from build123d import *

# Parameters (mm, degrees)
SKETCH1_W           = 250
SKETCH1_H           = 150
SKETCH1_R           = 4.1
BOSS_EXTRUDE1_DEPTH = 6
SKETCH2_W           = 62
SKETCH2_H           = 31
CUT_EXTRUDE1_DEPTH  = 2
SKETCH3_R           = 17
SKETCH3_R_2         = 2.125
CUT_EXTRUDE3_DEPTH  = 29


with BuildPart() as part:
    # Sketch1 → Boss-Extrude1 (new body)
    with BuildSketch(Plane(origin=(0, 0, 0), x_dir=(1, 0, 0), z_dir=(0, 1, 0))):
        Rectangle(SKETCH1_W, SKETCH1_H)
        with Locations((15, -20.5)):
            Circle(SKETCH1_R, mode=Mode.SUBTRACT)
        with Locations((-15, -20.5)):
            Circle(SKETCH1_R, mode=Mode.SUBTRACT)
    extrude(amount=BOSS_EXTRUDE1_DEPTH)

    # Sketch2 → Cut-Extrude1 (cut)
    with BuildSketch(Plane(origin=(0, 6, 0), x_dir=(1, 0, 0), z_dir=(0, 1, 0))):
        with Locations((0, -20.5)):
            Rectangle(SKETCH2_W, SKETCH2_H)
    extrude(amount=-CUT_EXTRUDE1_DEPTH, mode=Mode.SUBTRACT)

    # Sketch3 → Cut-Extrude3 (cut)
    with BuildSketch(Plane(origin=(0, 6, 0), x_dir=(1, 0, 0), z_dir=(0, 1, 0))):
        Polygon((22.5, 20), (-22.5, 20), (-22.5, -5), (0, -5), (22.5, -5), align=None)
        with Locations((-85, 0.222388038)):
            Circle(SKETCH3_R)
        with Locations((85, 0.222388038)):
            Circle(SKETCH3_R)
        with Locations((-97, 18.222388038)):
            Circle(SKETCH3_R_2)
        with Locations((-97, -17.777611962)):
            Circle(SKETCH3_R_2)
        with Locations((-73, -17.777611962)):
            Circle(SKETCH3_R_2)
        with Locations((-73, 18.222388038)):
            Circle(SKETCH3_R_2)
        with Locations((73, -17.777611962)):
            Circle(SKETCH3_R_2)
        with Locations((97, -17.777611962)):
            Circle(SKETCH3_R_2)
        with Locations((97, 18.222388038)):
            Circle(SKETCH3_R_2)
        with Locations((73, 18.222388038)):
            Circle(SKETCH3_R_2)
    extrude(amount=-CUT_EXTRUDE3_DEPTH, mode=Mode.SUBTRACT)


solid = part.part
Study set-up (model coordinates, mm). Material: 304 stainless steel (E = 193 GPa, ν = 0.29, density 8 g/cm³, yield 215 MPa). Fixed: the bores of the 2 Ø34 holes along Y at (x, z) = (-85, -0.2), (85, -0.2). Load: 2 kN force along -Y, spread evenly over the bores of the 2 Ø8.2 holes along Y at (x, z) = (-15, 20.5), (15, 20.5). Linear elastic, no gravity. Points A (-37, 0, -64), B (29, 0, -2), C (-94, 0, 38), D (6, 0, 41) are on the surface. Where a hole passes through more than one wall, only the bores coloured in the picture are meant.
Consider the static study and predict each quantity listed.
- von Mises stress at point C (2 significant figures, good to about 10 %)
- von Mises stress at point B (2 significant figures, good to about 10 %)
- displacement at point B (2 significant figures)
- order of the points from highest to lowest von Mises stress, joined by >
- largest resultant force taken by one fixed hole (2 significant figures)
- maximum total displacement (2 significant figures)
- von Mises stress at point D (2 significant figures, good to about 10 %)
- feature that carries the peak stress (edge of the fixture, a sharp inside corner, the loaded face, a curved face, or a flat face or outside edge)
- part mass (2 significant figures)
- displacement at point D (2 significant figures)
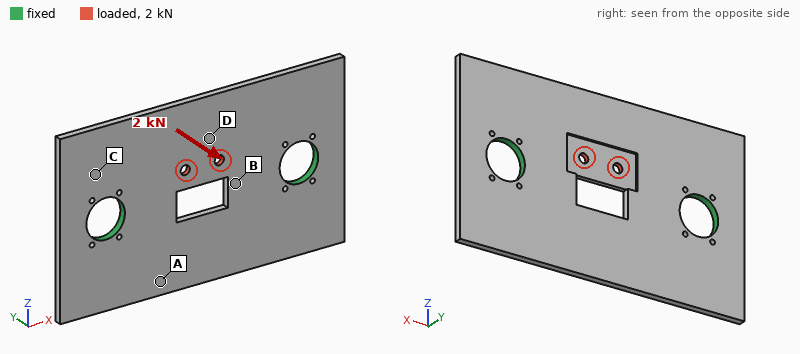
20 MPa
41 MPa
0.067 mm
D > B > C > A
1.3 kN
0.16 mm
54 MPa
the loaded face
1.6 kg
0.15 mm
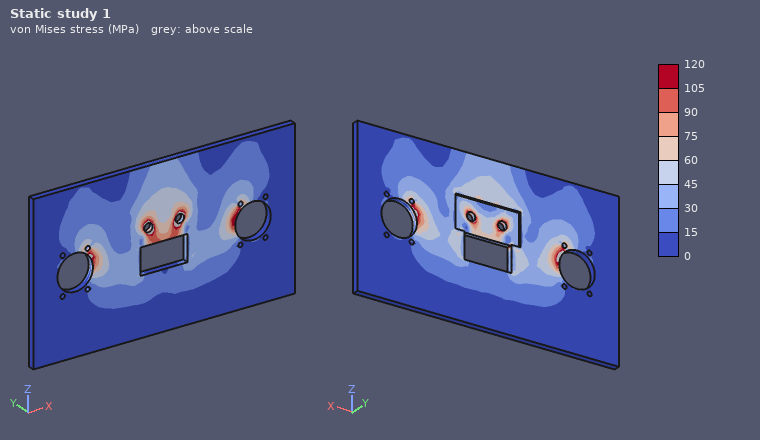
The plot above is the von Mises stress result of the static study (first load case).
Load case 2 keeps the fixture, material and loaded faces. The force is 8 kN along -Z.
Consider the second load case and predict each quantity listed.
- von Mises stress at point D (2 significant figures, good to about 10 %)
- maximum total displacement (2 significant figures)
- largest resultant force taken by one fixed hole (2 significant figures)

17 MPa
24 µm
4.1 kN
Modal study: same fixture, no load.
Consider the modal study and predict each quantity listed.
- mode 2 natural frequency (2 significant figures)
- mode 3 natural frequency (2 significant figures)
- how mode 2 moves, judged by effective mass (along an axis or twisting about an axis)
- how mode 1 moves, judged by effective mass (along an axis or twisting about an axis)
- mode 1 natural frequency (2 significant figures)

880 Hz
1300 Hz
along Y
twisting about X
820 Hz
